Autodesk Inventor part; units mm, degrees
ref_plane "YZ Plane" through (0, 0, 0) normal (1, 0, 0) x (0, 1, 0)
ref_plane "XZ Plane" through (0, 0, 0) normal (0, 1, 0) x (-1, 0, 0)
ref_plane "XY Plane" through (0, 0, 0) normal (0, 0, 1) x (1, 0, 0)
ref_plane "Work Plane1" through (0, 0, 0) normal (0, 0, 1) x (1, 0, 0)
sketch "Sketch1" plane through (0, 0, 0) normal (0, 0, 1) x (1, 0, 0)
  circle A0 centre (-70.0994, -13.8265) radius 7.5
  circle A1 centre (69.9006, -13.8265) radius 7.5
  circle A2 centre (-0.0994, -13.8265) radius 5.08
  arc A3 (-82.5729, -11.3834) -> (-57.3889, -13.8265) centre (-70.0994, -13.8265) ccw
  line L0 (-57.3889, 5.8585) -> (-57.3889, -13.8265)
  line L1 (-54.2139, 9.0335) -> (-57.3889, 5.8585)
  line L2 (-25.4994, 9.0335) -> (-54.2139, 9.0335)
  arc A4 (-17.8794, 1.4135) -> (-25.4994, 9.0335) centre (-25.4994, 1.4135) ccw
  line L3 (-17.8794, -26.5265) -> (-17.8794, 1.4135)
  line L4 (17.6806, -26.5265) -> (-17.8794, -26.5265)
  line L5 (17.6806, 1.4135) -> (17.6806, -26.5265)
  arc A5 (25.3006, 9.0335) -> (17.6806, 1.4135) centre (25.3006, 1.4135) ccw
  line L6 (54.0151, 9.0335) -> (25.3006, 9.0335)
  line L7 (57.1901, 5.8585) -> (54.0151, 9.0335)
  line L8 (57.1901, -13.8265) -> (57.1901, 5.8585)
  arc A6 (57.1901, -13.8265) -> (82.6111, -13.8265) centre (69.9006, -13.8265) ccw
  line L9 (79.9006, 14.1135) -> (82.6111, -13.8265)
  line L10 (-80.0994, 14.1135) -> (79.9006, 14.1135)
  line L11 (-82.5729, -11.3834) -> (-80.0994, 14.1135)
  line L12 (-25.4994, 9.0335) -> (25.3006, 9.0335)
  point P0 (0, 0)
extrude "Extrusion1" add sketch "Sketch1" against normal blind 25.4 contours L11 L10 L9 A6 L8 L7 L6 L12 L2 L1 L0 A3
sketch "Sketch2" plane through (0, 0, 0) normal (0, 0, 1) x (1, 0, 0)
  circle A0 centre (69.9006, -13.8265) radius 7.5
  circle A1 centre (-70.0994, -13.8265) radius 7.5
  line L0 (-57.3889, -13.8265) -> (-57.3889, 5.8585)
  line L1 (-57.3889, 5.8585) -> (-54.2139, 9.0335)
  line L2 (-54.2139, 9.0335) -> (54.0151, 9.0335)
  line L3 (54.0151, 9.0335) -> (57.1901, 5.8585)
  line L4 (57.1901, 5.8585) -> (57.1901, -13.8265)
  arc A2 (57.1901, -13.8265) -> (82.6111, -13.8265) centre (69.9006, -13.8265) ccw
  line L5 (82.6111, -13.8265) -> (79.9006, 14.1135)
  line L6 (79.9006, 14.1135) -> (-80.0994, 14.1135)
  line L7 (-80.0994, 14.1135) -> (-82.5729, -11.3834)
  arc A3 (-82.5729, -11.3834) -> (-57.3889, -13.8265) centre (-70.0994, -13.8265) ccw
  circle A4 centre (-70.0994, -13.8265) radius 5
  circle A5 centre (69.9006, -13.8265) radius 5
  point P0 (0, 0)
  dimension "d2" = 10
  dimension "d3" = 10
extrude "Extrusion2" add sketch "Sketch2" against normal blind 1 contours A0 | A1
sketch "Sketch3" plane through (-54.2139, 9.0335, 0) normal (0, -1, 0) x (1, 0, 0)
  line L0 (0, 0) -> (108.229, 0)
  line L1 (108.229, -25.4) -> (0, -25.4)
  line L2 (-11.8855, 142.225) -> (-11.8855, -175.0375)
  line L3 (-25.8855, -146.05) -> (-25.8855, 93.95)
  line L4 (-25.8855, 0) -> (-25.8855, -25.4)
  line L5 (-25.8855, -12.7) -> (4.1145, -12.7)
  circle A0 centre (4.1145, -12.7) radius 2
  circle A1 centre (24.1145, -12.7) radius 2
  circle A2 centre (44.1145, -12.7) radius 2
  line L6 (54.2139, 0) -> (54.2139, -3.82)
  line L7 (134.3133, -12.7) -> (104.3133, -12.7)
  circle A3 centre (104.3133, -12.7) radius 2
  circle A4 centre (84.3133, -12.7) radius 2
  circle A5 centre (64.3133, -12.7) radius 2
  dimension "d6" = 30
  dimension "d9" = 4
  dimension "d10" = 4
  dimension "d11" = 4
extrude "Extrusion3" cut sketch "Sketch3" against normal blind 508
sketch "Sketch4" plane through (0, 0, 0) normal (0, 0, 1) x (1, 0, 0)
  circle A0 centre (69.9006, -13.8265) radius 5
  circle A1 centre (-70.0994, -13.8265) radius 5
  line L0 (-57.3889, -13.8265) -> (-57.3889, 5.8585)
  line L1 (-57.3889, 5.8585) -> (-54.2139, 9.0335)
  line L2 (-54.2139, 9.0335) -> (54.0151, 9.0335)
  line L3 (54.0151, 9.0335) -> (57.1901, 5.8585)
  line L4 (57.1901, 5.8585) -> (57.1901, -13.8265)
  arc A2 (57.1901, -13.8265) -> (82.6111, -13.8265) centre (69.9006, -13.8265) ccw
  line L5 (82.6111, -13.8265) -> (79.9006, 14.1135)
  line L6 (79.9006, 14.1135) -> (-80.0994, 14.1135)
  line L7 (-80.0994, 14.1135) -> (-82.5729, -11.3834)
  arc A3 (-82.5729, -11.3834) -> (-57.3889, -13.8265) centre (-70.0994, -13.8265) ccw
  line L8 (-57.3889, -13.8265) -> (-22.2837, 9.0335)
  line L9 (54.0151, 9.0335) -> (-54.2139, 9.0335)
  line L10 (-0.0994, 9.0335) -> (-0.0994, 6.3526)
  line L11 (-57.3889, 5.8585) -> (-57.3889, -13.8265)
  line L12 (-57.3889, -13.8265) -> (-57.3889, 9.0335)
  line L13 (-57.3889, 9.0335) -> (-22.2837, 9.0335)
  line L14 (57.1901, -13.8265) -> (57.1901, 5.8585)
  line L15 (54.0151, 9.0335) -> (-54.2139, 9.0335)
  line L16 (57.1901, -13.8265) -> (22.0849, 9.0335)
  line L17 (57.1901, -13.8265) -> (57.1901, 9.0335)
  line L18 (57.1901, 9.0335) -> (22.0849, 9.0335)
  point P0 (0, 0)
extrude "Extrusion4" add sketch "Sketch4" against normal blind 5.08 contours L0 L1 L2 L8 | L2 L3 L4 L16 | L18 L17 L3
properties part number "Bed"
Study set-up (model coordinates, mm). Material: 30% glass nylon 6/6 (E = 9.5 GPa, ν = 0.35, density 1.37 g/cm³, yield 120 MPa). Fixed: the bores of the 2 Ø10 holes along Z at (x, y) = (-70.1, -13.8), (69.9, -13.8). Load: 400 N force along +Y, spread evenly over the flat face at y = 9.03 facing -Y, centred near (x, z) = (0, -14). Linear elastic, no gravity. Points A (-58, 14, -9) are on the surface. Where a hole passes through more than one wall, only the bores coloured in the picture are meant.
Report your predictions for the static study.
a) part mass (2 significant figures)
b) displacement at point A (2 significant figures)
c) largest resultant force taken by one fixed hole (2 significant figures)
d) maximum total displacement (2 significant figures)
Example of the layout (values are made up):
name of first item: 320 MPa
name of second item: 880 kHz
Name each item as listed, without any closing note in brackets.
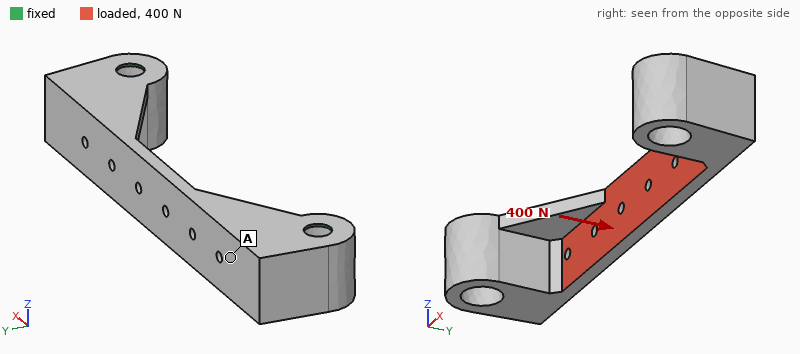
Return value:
part mass: 78 g
displacement at point A: 0.27 mm
largest resultant force taken by one fixed hole: 320 N
maximum total displacement: 0.67 mm
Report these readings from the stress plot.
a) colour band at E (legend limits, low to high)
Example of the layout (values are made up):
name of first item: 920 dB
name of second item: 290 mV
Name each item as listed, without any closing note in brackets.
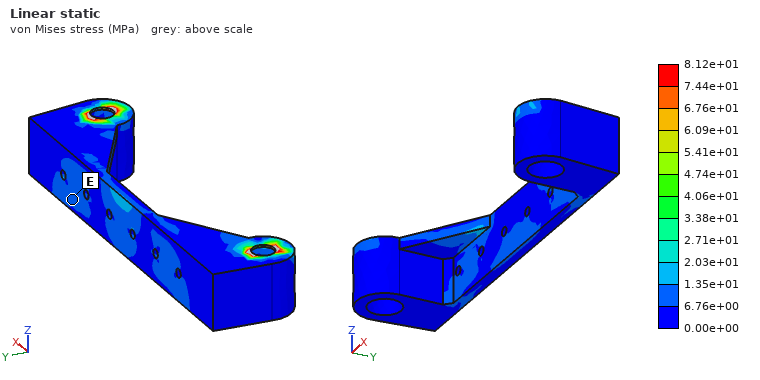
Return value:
colour band at E: 6.76e+00 to 1.35e+01 MPa
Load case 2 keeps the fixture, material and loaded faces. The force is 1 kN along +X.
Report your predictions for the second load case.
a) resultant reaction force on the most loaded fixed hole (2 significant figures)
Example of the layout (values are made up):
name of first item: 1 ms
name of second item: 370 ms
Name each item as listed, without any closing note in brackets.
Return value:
resultant reaction force on the most loaded fixed hole: 510 N
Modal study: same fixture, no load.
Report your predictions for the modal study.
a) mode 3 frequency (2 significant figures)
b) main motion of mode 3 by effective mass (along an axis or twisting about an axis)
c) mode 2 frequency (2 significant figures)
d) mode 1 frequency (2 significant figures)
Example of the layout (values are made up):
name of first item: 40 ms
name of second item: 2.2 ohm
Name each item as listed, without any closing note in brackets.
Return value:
mode 3 frequency: 1700 Hz
main motion of mode 3 by effective mass: along X
mode 2 frequency: 860 Hz
mode 1 frequency: 620 Hz
